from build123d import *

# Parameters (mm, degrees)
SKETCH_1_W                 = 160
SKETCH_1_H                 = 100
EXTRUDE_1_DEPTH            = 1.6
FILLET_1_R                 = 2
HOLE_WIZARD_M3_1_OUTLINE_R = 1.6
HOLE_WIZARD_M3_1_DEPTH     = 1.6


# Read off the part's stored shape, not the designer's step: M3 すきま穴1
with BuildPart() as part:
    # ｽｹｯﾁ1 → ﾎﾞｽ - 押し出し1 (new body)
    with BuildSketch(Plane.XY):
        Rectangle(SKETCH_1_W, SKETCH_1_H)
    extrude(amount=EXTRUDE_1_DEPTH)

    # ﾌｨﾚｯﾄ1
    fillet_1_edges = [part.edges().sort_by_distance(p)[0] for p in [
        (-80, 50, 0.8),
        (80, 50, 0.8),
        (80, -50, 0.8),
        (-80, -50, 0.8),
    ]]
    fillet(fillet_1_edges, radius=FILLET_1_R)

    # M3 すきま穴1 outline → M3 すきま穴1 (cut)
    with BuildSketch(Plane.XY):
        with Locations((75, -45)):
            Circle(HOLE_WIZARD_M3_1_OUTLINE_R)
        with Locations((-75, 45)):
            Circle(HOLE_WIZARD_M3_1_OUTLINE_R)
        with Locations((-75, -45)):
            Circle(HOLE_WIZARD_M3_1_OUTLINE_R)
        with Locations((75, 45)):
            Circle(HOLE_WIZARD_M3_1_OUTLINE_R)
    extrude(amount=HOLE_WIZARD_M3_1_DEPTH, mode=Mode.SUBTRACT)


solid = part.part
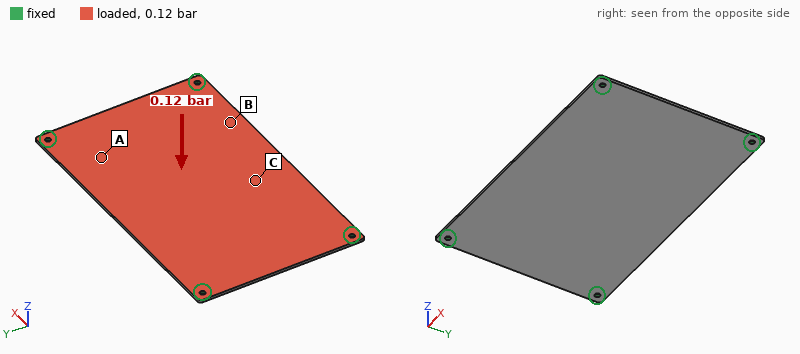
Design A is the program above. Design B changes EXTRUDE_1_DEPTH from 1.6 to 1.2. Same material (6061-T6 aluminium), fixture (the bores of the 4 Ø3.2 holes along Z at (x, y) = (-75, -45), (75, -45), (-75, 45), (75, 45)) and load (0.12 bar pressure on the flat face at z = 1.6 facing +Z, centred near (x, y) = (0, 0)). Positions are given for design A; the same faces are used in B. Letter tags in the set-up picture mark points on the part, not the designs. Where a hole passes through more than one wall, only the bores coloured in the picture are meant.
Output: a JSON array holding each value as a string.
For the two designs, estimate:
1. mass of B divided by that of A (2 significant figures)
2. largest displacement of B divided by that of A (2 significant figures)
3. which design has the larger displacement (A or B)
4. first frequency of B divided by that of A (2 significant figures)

["0.75", "2.3", "B", "0.75"]
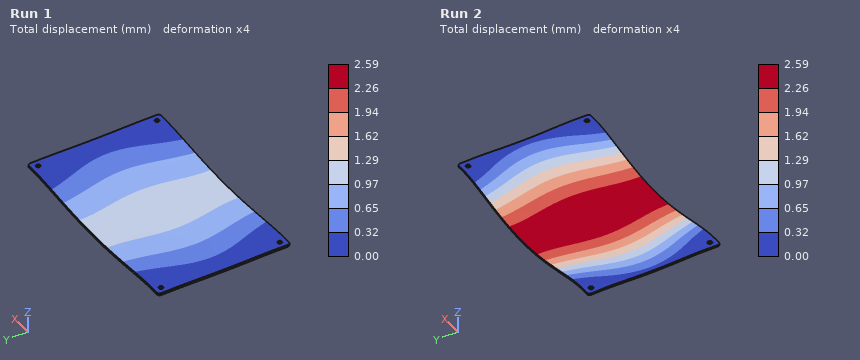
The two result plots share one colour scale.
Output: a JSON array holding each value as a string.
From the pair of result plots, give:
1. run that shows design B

["Run 2"]
